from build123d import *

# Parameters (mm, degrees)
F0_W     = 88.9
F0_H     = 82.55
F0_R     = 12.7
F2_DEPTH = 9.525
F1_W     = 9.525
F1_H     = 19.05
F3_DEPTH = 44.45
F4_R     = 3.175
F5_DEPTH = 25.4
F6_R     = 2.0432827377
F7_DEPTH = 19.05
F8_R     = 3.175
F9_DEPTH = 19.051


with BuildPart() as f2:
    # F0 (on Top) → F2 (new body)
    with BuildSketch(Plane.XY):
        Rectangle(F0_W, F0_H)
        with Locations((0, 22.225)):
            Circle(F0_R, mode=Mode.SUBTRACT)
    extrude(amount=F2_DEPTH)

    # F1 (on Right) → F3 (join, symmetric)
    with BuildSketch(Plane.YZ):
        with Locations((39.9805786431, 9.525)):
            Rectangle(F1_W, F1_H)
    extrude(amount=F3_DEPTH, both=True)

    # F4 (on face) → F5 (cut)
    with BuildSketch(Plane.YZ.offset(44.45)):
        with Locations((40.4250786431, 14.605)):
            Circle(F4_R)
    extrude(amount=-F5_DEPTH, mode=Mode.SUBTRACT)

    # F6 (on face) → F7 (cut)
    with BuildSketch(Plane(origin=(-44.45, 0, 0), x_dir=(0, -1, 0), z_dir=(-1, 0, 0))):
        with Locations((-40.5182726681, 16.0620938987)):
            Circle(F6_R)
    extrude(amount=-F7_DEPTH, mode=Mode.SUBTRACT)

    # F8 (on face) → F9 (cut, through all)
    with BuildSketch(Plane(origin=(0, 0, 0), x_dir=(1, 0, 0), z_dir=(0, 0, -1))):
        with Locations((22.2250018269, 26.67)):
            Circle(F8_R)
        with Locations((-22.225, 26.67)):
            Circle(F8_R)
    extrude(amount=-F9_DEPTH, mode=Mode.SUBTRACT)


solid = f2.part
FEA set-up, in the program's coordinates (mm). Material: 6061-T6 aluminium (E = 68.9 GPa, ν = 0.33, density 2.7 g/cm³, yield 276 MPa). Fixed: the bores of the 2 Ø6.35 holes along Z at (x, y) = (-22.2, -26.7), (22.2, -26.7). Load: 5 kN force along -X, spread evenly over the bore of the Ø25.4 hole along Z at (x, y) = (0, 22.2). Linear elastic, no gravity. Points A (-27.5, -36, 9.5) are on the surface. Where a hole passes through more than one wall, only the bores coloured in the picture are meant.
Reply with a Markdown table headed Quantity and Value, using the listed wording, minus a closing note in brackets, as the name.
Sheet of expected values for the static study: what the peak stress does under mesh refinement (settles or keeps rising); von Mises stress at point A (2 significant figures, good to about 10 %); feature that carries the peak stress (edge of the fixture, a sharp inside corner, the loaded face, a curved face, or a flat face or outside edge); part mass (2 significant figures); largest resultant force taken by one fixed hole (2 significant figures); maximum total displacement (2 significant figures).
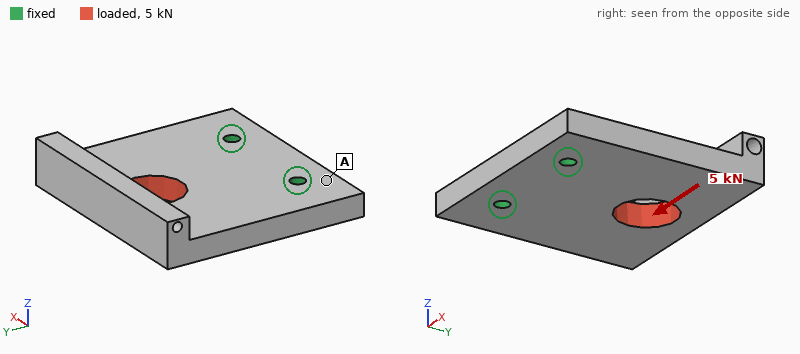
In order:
| Quantity | Value |
|---|---|
| what the peak stress does under mesh refinement | keeps rising |
| von Mises stress at point A | 13 MPa |
| feature that carries the peak stress | edge of the fixture |
| part mass | 200 g |
| largest resultant force taken by one fixed hole | 5.6 kN |
| maximum total displacement | 49 µm |
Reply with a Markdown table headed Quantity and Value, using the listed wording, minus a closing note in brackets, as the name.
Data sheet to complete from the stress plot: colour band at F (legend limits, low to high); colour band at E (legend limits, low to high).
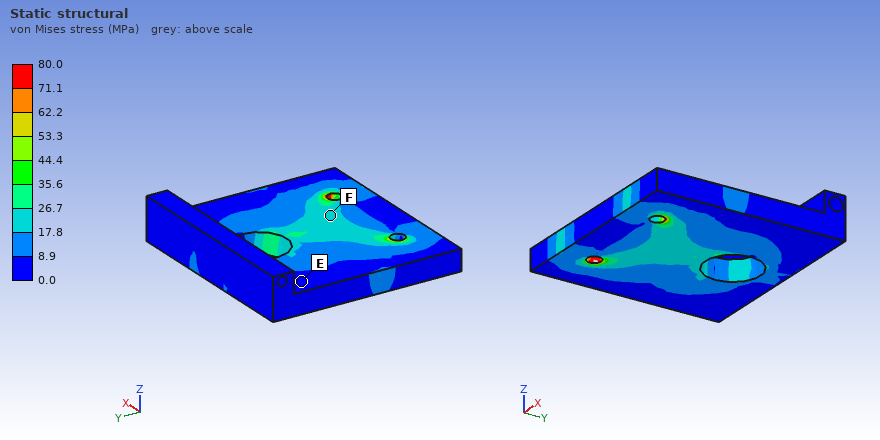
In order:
| Quantity | Value |
|---|---|
| colour band at F | 17.8 to 26.7 MPa |
| colour band at E | 0.0 to 8.9 MPa |
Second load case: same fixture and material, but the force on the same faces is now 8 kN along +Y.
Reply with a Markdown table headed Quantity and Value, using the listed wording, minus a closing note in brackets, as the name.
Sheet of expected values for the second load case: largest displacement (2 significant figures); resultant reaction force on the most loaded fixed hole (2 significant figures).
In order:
| Quantity | Value |
|---|---|
| largest displacement | 21 µm |
| resultant reaction force on the most loaded fixed hole | 4.0 kN |
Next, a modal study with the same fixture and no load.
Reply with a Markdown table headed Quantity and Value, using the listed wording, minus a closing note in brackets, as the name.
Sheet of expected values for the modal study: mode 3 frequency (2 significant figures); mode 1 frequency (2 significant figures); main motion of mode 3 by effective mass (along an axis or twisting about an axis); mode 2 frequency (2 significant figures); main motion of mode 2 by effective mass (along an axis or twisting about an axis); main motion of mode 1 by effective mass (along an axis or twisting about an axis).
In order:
| Quantity | Value |
|---|---|
| mode 3 frequency | 5100 Hz |
| mode 1 frequency | 1200 Hz |
| main motion of mode 3 by effective mass | along X |
| mode 2 frequency | 2400 Hz |
| main motion of mode 2 by effective mass | twisting about Y |
| main motion of mode 1 by effective mass | along Z |
